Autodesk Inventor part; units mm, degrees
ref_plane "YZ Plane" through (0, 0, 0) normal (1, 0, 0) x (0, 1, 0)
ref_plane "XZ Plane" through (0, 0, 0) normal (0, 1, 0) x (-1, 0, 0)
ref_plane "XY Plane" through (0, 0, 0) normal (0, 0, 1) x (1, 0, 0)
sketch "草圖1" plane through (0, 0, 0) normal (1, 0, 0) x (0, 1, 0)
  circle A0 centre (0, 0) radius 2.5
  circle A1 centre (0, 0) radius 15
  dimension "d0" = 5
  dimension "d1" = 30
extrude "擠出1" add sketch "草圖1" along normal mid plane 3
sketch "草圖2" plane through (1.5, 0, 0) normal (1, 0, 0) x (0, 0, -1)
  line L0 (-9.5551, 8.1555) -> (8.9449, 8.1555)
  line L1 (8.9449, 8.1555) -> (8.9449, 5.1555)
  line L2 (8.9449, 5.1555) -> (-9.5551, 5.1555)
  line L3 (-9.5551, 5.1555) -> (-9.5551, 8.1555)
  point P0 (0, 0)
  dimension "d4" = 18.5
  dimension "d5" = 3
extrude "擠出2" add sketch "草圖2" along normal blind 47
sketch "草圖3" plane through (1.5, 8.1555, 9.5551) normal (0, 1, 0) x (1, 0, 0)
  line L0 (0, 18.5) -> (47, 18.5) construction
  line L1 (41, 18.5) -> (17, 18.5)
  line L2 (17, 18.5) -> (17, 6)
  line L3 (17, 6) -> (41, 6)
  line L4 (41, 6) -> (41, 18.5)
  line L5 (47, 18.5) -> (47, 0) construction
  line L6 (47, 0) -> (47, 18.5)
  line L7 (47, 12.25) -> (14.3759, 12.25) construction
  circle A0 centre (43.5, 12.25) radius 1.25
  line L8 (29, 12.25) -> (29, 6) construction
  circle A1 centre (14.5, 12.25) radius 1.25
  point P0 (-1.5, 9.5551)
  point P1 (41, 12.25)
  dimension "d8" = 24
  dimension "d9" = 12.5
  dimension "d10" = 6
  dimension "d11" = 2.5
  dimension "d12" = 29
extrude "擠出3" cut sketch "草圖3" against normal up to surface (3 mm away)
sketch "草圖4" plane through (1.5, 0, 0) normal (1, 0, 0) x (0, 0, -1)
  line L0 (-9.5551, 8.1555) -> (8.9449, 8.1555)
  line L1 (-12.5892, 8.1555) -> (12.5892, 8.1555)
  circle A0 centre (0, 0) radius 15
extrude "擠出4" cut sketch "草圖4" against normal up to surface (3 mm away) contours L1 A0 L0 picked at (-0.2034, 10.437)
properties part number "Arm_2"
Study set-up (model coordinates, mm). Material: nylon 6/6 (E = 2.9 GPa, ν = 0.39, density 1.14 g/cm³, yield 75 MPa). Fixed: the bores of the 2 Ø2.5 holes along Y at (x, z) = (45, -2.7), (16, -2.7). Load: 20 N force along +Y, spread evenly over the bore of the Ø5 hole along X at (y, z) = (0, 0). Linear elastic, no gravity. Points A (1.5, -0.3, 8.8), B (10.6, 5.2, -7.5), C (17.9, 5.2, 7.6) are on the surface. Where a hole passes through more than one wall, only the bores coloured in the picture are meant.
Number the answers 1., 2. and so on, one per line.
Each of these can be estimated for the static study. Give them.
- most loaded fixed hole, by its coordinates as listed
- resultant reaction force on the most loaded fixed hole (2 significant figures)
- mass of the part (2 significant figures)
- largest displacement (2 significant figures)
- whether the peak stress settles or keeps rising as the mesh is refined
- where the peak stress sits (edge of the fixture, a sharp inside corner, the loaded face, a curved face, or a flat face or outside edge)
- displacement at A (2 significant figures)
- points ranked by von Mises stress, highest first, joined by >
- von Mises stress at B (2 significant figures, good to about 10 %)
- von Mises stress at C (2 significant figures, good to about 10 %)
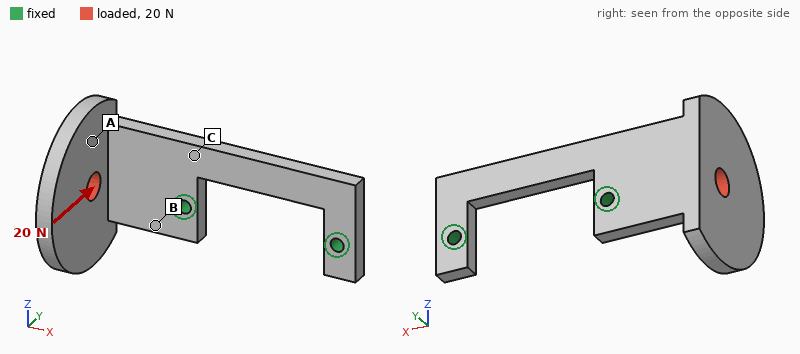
1. (16, -2.7)
2. 22 N
3. 3.8 g
4. 0.62 mm
5. keeps rising
6. edge of the fixture
7. 0.32 mm
8. B > C > A
9. 8.1 MPa
10. 4.4 MPa
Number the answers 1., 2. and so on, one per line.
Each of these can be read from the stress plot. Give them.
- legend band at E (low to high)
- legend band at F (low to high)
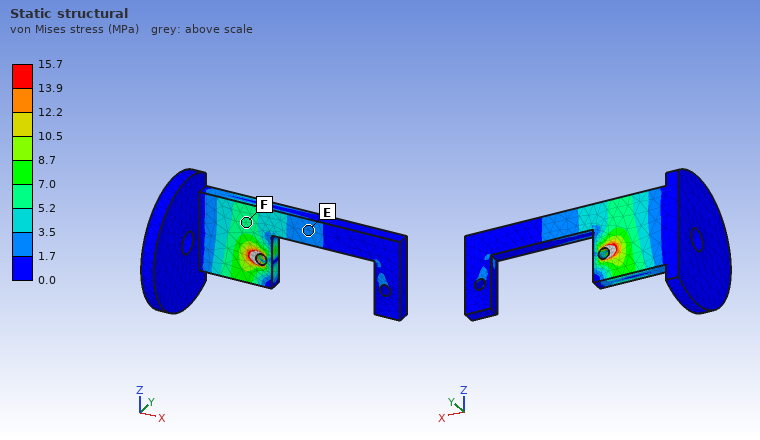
1. 1.7 to 3.5 MPa
2. 5.2 to 7.0 MPa
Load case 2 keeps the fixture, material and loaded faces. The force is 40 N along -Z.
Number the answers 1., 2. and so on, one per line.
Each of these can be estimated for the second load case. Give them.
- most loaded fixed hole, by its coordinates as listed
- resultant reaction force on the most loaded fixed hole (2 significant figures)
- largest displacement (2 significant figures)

1. (16, -2.7)
2. 53 N
3. 0.68 mm
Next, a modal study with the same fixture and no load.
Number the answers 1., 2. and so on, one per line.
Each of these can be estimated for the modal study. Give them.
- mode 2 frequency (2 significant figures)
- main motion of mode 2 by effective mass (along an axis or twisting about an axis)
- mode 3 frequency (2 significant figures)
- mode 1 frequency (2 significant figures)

1. 810 Hz
2. along Z
3. 1900 Hz
4. 640 Hz
